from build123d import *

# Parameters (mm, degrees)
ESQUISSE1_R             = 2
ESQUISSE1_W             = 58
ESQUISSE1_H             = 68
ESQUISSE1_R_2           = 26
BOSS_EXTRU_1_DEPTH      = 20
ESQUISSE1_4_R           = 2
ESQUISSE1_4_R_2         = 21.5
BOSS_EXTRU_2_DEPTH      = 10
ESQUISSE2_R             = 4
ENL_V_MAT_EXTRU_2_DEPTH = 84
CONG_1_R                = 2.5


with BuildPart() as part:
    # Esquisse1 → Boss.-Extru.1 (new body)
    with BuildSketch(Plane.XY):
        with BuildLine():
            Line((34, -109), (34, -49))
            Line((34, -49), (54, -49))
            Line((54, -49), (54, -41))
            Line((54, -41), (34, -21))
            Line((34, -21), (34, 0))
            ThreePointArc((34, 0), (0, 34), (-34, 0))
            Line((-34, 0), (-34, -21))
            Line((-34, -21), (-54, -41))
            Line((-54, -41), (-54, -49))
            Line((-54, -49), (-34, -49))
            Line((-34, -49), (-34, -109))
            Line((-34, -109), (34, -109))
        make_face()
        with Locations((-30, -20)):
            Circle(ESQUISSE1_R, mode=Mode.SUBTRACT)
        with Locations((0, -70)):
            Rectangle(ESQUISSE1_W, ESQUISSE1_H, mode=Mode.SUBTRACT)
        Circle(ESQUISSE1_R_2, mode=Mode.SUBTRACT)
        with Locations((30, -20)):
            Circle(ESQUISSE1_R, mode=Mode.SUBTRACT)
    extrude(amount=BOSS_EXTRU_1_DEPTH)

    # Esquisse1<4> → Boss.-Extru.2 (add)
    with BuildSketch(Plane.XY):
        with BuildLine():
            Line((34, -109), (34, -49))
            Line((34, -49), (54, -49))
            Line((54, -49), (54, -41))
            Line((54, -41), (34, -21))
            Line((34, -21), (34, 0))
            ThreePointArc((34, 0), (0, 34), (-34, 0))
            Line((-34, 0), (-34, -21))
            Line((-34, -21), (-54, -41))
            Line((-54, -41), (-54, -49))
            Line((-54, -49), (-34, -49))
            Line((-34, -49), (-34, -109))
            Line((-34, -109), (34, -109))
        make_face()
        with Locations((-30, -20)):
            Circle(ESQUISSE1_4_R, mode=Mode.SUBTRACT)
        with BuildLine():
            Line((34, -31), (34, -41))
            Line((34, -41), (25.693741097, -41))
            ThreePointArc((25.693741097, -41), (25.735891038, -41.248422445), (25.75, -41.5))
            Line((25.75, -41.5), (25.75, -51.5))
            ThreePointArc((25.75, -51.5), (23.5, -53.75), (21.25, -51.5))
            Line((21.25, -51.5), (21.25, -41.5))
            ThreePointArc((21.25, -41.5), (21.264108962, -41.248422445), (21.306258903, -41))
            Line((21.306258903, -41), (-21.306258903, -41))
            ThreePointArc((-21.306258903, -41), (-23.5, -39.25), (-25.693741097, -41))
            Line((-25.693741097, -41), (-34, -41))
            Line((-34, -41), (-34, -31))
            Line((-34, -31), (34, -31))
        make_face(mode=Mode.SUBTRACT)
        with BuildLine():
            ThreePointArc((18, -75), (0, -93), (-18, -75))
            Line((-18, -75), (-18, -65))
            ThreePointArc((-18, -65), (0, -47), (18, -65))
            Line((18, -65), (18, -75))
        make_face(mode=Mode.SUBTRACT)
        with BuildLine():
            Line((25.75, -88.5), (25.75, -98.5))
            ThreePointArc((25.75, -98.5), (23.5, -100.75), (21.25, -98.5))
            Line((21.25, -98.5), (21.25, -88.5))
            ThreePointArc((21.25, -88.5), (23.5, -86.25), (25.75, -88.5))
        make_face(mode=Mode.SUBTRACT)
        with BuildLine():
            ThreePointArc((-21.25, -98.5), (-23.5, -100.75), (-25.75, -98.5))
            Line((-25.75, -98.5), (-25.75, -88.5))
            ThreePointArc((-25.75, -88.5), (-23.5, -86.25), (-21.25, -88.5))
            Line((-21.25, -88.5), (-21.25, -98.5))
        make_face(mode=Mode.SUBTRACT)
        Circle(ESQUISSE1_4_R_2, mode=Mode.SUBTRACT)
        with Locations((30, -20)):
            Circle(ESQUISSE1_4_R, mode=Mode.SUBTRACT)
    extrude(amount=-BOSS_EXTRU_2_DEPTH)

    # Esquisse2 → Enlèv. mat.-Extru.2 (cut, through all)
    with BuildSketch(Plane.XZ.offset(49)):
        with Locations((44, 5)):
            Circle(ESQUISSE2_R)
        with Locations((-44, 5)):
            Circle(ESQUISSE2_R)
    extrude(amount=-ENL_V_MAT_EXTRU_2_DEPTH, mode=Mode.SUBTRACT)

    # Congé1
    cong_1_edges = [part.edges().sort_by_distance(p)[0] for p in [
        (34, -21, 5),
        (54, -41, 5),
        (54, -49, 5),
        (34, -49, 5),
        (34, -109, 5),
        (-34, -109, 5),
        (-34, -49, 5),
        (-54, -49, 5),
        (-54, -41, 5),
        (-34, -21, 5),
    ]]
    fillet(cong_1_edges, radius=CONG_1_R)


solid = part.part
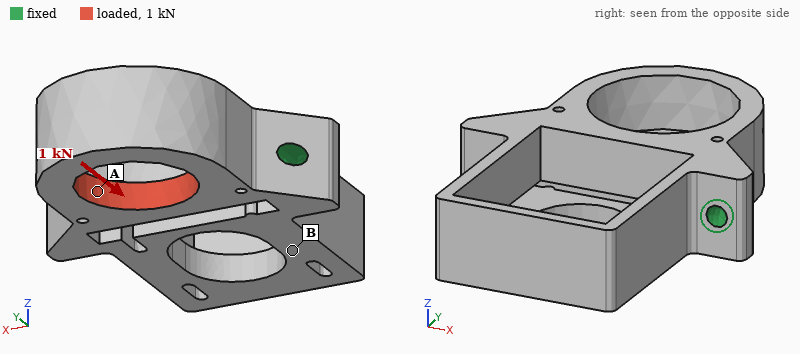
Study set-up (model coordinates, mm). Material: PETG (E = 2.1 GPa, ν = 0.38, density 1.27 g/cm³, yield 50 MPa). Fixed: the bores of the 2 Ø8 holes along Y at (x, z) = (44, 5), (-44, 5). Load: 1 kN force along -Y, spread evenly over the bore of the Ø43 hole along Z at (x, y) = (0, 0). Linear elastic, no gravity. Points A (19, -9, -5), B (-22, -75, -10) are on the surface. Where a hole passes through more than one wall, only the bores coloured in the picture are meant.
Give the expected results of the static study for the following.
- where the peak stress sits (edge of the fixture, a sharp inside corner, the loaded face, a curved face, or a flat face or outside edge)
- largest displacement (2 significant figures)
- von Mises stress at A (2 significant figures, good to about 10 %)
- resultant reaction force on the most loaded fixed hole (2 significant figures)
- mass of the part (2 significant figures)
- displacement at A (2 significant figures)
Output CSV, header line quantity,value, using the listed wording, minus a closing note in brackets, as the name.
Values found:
quantity,value
where the peak stress sits,a curved face
largest displacement,0.39 mm
von Mises stress at A,2.0 MPa
resultant reaction force on the most loaded fixed hole,560 N
mass of the part,170 g
displacement at A,0.15 mm
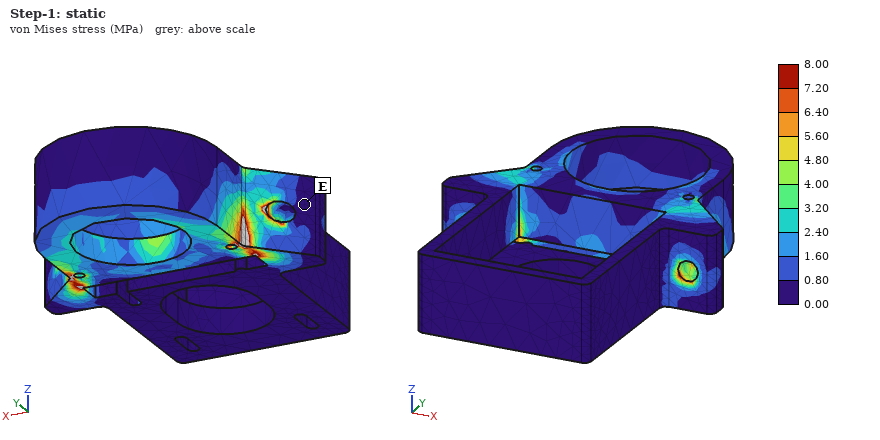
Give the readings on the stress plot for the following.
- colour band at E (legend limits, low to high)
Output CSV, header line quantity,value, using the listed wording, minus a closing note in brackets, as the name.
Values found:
quantity,value
colour band at E,0.00 to 0.80 MPa
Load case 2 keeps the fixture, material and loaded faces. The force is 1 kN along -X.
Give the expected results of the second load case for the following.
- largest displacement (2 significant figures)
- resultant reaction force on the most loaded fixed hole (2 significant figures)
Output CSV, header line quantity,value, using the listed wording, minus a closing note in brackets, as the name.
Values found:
quantity,value
largest displacement,0.36 mm
resultant reaction force on the most loaded fixed hole,650 N
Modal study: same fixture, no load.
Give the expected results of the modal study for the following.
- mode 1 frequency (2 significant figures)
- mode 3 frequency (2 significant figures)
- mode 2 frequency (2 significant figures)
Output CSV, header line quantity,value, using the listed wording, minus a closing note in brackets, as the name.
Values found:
quantity,value
mode 1 frequency,560 Hz
mode 3 frequency,730 Hz
mode 2 frequency,720 Hz
